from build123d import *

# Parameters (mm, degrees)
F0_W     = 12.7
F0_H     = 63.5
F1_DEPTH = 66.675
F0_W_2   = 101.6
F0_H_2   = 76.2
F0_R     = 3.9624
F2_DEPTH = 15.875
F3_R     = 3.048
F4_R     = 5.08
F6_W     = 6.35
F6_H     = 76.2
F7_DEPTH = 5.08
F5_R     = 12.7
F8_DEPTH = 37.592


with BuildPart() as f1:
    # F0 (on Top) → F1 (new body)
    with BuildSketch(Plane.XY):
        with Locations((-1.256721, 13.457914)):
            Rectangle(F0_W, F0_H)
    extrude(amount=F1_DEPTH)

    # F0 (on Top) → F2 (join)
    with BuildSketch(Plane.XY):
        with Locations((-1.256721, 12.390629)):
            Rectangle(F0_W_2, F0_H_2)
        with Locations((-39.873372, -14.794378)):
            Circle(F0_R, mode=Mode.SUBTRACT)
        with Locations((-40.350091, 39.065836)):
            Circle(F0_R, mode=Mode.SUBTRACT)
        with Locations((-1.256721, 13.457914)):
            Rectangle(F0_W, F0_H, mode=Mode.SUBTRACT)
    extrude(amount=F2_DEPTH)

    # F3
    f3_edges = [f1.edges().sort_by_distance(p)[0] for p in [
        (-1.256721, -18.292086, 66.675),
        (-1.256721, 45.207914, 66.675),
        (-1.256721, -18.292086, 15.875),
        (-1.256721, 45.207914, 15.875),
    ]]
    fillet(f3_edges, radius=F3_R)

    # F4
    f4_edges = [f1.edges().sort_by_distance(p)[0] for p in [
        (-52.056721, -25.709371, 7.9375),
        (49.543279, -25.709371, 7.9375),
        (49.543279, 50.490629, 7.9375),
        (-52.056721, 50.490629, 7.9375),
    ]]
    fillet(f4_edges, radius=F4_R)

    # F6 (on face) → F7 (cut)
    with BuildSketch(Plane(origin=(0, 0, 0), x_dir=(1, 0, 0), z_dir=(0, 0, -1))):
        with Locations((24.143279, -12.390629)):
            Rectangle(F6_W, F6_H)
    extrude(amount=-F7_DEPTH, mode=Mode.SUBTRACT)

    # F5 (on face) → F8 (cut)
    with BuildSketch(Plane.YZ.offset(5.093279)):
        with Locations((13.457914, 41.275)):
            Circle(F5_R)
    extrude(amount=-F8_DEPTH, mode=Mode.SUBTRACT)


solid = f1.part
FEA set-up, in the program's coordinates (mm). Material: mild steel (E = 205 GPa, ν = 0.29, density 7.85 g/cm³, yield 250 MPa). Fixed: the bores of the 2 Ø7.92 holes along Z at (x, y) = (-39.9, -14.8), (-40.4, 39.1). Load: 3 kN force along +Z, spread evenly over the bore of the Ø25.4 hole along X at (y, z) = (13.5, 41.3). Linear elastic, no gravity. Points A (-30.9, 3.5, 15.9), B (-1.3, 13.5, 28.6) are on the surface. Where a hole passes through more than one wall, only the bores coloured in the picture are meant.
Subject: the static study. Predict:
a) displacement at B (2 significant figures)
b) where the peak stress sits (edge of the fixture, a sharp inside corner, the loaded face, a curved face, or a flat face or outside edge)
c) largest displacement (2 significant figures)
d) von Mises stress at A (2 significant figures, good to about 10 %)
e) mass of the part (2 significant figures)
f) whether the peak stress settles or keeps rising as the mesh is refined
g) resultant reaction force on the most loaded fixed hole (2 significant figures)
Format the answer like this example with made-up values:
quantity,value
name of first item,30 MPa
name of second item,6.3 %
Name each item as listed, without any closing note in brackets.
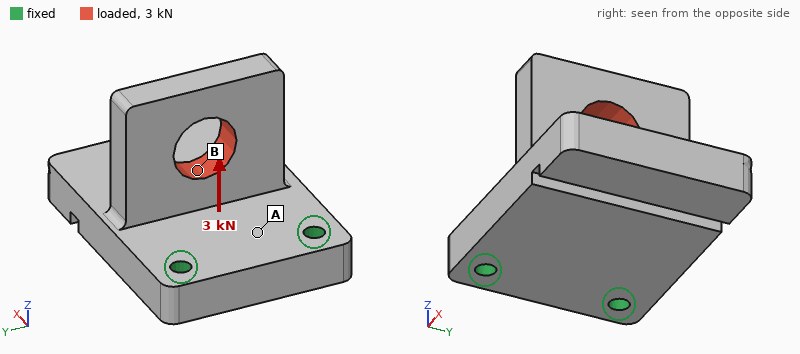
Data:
quantity,value
displacement at B,19 µm
where the peak stress sits,edge of the fixture
largest displacement,42 µm
von Mises stress at A,16 MPa
mass of the part,1.2 kg
whether the peak stress settles or keeps rising as the mesh is refined,keeps rising
resultant reaction force on the most loaded fixed hole,1.5 kN
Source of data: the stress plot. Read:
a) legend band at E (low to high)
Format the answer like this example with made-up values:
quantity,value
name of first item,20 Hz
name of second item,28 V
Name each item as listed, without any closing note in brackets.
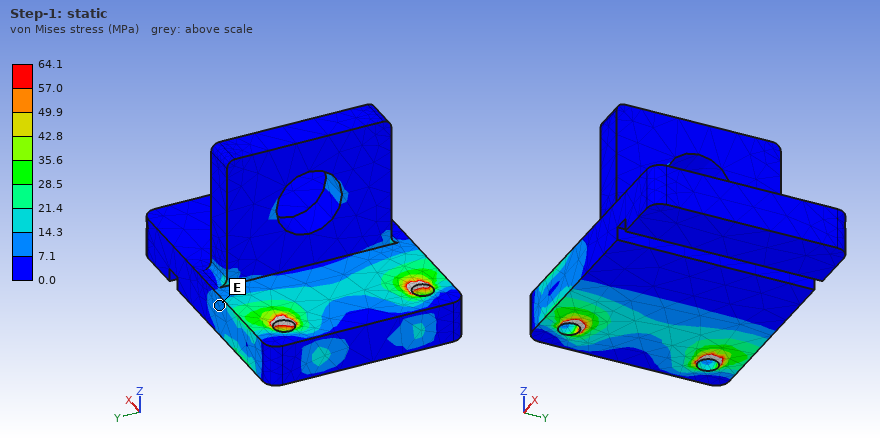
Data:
quantity,value
legend band at E,7.1 to 14.3 MPa
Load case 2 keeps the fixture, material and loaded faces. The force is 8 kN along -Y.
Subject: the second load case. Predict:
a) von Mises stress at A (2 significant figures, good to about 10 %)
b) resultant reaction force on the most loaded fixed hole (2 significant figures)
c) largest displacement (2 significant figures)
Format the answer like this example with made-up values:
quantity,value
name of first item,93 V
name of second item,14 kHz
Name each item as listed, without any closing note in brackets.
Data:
quantity,value
von Mises stress at A,40 MPa
resultant reaction force on the most loaded fixed hole,8.0 kN
largest displacement,58 µm
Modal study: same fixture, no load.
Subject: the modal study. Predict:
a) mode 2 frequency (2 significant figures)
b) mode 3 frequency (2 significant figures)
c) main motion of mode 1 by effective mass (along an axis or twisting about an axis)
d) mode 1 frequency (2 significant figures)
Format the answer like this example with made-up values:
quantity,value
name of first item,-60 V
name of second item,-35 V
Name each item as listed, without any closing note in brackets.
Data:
quantity,value
mode 2 frequency,3200 Hz
mode 3 frequency,3400 Hz
main motion of mode 1 by effective mass,along Z
mode 1 frequency,1300 Hz
